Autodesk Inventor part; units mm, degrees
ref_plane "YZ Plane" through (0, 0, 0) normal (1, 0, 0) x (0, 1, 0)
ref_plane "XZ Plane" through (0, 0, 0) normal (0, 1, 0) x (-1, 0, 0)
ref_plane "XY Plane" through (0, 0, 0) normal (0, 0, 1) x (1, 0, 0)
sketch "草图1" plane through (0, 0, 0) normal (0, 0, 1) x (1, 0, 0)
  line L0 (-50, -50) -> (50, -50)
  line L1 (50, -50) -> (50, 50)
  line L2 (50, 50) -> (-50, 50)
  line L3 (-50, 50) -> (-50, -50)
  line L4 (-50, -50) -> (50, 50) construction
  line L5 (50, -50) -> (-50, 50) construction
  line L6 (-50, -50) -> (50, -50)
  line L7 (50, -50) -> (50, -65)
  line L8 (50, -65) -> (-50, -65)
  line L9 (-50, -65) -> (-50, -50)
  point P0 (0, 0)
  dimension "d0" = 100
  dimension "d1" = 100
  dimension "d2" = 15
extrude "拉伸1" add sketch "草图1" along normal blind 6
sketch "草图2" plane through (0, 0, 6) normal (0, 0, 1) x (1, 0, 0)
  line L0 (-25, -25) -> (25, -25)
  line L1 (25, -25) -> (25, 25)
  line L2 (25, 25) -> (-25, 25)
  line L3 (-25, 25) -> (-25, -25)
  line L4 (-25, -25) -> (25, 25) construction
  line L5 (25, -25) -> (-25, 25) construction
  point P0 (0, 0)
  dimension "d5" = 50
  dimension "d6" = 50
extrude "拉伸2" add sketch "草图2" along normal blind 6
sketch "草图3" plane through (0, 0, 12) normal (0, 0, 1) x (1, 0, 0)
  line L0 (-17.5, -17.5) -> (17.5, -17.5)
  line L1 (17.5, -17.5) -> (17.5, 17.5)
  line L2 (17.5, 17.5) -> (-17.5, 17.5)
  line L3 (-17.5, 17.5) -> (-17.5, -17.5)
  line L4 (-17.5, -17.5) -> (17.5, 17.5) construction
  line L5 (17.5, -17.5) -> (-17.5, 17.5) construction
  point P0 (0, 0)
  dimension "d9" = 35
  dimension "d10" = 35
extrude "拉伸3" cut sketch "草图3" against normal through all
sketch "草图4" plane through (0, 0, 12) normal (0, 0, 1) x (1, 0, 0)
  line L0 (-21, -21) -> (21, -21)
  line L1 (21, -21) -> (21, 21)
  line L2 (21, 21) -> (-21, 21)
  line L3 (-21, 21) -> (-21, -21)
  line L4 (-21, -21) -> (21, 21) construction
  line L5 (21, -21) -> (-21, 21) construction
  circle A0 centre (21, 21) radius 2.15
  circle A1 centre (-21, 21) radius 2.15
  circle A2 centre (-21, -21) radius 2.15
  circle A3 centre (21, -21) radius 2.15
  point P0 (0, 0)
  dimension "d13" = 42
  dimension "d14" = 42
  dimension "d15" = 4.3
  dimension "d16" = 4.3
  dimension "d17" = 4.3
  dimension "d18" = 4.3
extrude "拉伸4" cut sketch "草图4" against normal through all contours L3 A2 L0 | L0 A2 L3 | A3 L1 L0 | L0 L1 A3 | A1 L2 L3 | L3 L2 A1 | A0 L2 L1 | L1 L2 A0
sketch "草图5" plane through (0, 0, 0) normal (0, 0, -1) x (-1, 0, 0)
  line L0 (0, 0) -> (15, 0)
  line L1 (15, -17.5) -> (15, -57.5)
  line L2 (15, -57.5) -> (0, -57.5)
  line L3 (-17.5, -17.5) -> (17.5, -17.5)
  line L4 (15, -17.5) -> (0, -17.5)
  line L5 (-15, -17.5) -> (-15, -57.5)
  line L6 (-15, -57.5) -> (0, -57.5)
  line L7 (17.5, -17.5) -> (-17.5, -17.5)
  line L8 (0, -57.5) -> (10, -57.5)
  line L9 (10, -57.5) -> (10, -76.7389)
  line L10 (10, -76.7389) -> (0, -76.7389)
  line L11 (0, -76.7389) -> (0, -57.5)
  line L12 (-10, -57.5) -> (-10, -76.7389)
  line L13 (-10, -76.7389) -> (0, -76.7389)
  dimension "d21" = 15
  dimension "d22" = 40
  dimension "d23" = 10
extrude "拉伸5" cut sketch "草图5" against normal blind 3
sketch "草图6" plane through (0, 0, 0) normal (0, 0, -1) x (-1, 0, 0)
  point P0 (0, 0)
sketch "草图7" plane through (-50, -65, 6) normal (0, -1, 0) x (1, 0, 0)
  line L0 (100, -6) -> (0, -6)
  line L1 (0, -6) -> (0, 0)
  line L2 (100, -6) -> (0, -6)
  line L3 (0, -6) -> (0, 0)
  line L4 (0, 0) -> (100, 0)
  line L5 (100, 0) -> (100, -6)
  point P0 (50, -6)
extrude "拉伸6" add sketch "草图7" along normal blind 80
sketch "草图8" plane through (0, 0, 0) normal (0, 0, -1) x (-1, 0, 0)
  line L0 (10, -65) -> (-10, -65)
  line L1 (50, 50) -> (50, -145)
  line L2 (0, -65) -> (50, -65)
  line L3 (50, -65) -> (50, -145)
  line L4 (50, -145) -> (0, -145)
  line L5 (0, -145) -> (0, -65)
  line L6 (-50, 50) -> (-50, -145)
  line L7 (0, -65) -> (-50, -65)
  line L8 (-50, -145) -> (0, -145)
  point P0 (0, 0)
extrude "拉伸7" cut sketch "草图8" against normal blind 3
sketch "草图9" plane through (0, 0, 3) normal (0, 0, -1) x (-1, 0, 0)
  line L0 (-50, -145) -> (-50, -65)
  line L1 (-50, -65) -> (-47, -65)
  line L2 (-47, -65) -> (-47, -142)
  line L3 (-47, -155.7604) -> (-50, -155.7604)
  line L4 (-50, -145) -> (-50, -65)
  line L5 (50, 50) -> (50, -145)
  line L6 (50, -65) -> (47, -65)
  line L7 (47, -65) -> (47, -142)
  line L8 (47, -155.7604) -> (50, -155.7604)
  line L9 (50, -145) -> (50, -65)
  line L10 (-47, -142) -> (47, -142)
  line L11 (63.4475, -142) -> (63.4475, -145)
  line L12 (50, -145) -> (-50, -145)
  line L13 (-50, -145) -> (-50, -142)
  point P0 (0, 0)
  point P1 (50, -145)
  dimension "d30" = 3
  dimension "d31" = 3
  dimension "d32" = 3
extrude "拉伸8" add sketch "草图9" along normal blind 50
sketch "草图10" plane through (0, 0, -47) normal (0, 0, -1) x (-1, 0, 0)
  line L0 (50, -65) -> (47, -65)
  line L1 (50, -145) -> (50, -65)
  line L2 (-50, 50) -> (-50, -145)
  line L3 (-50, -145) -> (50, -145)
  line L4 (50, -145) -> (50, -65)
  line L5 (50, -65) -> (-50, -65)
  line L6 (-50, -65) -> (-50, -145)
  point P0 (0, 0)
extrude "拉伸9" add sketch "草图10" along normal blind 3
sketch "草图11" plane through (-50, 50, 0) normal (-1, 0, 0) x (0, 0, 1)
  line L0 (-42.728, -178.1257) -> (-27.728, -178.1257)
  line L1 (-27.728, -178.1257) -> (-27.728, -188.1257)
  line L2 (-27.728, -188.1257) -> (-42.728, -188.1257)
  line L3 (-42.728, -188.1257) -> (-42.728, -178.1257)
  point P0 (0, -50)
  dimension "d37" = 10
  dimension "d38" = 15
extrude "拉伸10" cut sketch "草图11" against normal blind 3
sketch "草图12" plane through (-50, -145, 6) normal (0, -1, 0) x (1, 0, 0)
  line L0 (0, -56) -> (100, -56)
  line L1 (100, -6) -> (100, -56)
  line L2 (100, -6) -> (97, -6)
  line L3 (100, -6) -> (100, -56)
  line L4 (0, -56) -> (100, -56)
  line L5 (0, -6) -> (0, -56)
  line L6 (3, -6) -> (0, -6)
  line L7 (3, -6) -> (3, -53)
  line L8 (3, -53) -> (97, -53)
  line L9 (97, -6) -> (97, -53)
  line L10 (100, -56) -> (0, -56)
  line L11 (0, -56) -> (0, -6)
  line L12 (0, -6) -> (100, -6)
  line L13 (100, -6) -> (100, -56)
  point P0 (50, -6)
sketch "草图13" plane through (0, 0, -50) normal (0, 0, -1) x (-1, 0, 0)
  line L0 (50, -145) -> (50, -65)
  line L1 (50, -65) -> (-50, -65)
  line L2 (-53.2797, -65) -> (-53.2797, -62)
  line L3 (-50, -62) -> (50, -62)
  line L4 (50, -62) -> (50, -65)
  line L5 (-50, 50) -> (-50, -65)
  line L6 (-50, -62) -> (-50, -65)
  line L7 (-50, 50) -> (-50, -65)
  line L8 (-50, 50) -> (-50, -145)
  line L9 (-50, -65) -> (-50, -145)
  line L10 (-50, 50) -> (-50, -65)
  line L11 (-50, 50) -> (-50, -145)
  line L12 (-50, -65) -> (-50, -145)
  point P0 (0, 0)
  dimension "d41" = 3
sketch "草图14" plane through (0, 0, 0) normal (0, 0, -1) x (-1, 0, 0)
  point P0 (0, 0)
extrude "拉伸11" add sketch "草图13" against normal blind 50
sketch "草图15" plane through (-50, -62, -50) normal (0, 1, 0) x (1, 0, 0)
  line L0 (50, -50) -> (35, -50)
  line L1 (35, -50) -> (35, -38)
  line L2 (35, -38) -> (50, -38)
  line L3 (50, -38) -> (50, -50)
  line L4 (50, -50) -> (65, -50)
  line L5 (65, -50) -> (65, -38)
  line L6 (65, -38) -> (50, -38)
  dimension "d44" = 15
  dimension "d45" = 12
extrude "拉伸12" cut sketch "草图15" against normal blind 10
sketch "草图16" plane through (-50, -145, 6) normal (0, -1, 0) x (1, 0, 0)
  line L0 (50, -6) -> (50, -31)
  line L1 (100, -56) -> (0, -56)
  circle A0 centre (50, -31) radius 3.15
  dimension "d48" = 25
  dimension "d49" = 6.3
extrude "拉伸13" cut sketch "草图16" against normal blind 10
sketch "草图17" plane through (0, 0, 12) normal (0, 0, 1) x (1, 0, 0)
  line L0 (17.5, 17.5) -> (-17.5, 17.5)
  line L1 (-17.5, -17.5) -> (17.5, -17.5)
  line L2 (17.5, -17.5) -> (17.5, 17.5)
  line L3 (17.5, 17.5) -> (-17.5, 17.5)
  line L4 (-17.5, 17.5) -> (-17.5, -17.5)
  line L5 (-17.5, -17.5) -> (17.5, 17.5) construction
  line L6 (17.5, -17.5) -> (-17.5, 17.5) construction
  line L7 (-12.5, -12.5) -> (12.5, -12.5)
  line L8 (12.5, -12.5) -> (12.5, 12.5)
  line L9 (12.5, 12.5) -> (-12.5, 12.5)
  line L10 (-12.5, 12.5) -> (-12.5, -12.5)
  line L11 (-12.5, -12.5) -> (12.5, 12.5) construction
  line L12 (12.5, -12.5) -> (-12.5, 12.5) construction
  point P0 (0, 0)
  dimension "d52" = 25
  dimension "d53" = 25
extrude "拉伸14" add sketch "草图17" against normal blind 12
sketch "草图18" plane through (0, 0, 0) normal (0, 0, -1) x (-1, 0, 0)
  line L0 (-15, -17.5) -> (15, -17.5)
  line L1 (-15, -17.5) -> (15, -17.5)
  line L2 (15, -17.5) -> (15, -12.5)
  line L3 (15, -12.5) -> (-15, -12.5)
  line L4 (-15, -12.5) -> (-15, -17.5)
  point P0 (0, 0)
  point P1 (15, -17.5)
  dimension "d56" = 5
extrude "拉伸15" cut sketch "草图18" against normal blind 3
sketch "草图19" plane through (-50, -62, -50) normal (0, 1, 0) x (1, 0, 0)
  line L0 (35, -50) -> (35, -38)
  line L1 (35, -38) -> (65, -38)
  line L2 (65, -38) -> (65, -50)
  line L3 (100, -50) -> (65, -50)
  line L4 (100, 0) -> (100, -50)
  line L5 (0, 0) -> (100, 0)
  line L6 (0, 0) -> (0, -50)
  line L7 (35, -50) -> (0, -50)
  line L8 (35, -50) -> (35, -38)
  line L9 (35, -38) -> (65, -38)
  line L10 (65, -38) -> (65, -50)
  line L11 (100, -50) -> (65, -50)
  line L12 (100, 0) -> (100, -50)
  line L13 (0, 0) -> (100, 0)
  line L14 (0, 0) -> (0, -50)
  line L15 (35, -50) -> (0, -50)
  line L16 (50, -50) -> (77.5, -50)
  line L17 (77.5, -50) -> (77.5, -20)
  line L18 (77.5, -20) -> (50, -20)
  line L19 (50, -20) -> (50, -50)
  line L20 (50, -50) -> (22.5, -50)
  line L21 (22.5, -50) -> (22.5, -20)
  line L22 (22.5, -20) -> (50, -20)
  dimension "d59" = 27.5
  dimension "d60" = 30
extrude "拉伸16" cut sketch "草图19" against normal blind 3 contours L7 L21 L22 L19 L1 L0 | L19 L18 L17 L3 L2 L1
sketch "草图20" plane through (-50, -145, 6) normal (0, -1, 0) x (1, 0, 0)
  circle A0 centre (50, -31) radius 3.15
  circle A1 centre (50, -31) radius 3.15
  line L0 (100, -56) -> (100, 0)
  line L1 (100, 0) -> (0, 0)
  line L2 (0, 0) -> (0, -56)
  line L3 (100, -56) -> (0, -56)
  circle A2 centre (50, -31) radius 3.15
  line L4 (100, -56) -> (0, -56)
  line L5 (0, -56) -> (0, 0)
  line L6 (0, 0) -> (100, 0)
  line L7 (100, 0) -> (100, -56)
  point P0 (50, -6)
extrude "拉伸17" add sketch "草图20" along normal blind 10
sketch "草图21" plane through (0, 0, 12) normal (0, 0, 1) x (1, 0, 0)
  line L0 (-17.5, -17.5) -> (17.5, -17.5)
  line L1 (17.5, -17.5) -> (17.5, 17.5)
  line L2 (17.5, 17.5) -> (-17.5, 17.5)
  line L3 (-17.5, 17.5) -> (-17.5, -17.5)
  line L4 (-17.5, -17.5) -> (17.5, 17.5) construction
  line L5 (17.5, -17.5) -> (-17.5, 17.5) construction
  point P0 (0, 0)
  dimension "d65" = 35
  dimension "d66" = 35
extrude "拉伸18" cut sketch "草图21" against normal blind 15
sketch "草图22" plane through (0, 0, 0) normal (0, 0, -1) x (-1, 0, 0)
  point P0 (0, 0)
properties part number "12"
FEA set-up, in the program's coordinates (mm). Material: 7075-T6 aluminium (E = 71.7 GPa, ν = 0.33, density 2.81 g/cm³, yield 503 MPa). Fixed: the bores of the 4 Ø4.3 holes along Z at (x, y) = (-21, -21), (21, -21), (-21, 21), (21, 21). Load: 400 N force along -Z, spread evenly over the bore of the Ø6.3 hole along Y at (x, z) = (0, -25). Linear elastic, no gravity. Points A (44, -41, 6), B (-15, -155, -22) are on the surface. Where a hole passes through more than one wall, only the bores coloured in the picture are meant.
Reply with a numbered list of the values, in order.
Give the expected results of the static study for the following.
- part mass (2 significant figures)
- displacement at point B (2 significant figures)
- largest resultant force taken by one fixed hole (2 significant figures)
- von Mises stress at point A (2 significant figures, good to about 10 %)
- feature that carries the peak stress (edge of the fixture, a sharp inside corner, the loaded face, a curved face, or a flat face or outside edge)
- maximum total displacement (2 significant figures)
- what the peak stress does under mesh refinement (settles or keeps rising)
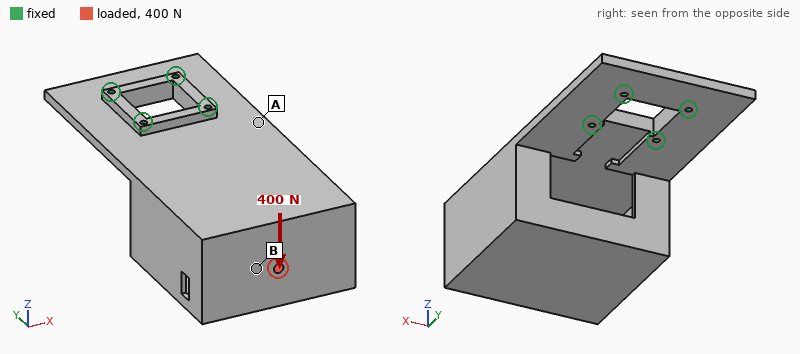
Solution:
1. 610 g
2. 2.6 mm
3. 890 N
4. 81 MPa
5. edge of the fixture
6. 2.8 mm
7. keeps rising
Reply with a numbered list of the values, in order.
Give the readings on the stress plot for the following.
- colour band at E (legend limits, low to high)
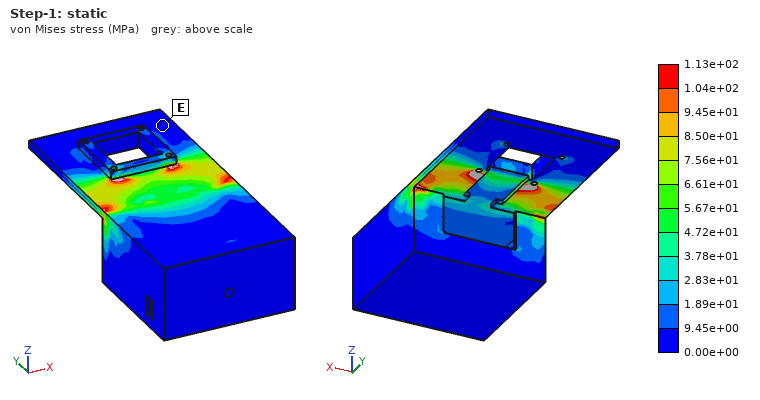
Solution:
1. 0.00e+00 to 9.45e+00 MPa
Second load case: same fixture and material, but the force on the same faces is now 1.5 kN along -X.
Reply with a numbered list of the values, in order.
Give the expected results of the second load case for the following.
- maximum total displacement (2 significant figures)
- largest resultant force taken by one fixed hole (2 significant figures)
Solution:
1. 0.45 mm
2. 2.4 kN
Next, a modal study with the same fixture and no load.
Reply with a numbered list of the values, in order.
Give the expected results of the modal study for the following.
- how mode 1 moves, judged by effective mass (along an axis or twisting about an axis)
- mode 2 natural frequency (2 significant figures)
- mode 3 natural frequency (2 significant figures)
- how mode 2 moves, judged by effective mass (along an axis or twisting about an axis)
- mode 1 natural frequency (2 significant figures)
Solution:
1. along Z
2. 470 Hz
3. 1100 Hz
4. along X
5. 120 Hz
